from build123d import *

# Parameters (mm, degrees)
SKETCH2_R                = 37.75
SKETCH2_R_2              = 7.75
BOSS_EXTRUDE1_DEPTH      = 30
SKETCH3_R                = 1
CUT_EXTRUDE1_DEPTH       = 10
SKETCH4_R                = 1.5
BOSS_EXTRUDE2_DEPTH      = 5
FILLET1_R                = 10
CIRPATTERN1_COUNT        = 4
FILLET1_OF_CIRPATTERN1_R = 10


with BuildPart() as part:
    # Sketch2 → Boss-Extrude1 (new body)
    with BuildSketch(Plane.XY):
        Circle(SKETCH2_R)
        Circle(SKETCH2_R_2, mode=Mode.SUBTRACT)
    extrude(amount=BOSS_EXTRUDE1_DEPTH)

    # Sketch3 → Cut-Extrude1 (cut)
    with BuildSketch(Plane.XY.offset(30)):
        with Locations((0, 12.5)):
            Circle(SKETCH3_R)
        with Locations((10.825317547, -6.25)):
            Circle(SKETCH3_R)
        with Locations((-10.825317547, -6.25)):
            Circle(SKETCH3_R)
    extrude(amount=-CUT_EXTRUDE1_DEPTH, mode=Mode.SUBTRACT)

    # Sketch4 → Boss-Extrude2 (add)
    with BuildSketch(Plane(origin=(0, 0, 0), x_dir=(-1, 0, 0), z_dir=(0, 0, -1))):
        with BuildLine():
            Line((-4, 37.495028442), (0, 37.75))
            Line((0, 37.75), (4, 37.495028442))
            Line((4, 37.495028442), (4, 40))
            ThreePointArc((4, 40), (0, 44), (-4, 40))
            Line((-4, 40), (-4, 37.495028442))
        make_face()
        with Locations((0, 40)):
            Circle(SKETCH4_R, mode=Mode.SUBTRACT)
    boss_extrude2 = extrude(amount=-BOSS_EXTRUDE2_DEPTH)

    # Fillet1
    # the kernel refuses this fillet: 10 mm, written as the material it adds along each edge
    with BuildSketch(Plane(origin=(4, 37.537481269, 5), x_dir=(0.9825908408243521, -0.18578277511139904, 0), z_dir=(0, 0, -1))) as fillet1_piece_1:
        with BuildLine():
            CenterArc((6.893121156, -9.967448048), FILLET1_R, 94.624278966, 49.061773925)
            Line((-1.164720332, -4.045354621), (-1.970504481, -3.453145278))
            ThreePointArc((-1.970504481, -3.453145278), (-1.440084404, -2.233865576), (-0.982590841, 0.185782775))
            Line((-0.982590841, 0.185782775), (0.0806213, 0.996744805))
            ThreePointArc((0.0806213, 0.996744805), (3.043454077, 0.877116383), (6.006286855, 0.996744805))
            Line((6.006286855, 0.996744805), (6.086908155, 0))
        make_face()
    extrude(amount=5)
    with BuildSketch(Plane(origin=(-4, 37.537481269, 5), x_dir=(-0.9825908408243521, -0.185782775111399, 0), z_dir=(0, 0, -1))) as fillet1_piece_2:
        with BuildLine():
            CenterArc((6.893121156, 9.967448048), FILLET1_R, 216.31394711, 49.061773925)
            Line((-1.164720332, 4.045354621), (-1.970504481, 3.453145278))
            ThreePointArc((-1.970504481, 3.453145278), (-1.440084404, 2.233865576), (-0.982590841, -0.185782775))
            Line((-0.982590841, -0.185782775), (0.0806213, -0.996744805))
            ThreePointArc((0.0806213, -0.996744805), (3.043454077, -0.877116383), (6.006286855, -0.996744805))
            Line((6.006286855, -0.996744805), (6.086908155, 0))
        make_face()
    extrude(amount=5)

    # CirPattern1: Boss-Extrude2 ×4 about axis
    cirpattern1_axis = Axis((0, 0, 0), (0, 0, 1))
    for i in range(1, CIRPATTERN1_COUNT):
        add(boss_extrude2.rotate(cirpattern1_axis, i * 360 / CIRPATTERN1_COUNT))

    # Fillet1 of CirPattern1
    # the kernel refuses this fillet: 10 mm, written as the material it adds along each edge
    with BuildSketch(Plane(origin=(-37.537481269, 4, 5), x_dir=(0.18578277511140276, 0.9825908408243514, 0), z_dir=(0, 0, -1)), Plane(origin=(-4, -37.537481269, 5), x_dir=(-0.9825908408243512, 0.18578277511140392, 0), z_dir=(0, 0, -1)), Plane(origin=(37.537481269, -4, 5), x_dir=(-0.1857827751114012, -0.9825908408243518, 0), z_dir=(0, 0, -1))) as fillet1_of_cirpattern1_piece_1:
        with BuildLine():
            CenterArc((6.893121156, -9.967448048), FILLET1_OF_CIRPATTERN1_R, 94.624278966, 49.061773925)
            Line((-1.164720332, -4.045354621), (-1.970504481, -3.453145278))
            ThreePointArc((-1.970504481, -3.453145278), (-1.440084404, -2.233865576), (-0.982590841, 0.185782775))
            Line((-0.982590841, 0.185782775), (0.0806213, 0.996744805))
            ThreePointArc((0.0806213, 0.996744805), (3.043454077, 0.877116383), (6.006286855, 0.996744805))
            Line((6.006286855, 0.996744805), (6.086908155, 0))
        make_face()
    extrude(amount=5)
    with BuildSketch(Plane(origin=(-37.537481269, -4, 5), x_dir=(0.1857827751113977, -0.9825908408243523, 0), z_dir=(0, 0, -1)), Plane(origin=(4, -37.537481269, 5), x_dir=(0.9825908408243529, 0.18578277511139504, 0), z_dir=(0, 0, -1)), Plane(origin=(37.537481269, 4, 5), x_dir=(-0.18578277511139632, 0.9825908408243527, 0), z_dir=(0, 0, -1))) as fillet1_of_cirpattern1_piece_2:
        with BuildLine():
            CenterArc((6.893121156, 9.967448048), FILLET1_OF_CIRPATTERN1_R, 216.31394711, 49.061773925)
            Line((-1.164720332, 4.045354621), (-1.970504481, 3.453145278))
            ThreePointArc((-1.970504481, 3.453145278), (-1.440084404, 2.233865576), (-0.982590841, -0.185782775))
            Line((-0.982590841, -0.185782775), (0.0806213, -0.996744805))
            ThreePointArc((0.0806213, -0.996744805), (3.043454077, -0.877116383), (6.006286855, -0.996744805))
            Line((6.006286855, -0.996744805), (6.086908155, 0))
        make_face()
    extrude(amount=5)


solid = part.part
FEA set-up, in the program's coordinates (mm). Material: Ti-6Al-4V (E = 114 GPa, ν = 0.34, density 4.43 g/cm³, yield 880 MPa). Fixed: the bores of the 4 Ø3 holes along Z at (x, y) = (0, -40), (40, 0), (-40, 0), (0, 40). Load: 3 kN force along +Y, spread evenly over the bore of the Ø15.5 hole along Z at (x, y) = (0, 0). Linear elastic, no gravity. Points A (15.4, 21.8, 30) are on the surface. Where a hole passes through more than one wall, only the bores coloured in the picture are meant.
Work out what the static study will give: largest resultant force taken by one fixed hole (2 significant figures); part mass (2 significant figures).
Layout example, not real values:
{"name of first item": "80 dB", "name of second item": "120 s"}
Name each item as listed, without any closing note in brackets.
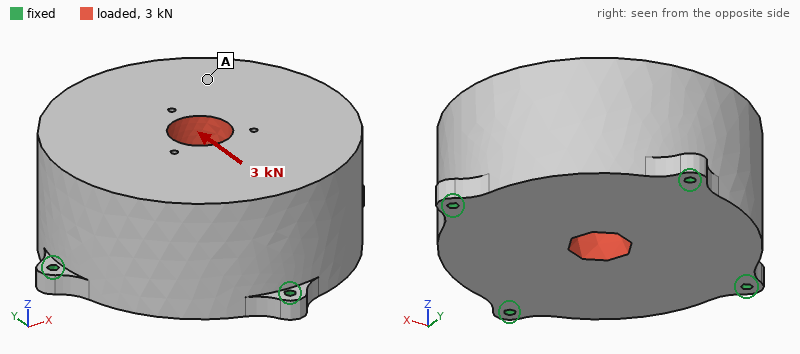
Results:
{"largest resultant force taken by one fixed hole": "1.1 kN", "part mass": "570 g"}
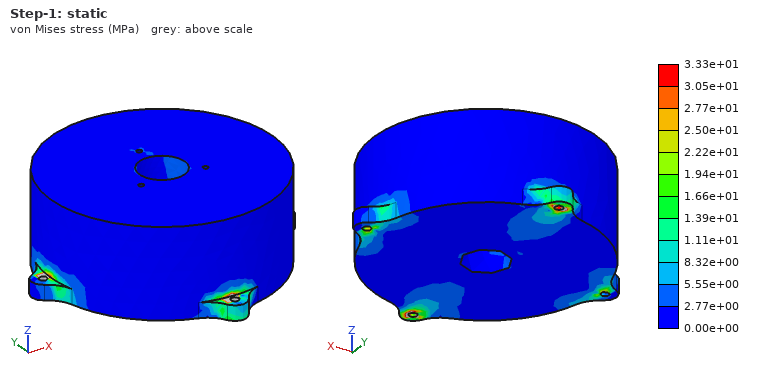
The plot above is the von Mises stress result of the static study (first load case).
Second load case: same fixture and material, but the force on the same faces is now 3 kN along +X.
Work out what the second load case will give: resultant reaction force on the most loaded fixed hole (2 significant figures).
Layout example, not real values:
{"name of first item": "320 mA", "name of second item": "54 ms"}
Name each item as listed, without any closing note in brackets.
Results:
{"resultant reaction force on the most loaded fixed hole": "1.1 kN"}
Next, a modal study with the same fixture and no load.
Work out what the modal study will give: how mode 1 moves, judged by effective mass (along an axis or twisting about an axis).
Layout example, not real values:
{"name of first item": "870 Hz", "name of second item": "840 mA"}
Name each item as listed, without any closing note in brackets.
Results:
{"how mode 1 moves, judged by effective mass": "along Z"}
